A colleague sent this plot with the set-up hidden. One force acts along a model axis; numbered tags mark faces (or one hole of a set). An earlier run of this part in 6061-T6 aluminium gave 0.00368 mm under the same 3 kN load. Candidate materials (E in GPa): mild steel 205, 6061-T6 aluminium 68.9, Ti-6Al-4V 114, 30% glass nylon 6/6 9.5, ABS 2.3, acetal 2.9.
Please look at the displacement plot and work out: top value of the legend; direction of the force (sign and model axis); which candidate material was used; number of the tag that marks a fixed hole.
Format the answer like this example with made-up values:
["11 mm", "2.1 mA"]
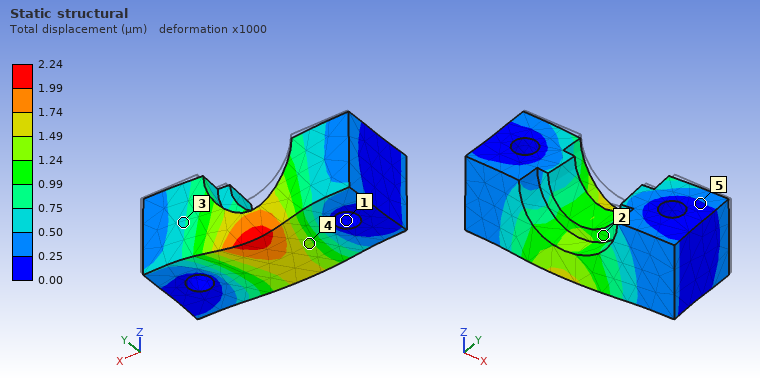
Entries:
["2.24 µm", "-Y", "Ti-6Al-4V", "1"]
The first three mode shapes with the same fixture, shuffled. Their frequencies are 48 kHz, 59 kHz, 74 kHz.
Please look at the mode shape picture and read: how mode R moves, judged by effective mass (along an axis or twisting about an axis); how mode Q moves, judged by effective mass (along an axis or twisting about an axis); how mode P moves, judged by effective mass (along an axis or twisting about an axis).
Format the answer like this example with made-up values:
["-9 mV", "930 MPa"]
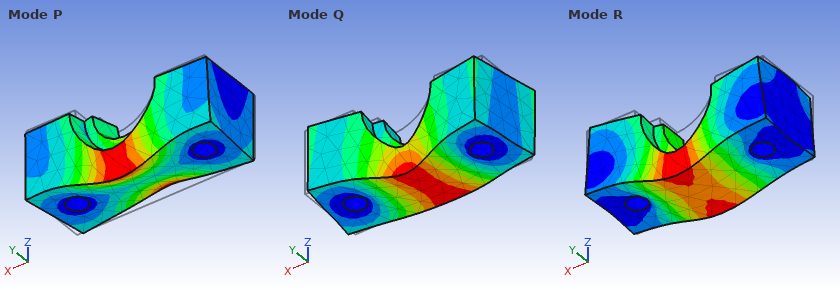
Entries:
["along Z", "along Y", "twisting about X"]
